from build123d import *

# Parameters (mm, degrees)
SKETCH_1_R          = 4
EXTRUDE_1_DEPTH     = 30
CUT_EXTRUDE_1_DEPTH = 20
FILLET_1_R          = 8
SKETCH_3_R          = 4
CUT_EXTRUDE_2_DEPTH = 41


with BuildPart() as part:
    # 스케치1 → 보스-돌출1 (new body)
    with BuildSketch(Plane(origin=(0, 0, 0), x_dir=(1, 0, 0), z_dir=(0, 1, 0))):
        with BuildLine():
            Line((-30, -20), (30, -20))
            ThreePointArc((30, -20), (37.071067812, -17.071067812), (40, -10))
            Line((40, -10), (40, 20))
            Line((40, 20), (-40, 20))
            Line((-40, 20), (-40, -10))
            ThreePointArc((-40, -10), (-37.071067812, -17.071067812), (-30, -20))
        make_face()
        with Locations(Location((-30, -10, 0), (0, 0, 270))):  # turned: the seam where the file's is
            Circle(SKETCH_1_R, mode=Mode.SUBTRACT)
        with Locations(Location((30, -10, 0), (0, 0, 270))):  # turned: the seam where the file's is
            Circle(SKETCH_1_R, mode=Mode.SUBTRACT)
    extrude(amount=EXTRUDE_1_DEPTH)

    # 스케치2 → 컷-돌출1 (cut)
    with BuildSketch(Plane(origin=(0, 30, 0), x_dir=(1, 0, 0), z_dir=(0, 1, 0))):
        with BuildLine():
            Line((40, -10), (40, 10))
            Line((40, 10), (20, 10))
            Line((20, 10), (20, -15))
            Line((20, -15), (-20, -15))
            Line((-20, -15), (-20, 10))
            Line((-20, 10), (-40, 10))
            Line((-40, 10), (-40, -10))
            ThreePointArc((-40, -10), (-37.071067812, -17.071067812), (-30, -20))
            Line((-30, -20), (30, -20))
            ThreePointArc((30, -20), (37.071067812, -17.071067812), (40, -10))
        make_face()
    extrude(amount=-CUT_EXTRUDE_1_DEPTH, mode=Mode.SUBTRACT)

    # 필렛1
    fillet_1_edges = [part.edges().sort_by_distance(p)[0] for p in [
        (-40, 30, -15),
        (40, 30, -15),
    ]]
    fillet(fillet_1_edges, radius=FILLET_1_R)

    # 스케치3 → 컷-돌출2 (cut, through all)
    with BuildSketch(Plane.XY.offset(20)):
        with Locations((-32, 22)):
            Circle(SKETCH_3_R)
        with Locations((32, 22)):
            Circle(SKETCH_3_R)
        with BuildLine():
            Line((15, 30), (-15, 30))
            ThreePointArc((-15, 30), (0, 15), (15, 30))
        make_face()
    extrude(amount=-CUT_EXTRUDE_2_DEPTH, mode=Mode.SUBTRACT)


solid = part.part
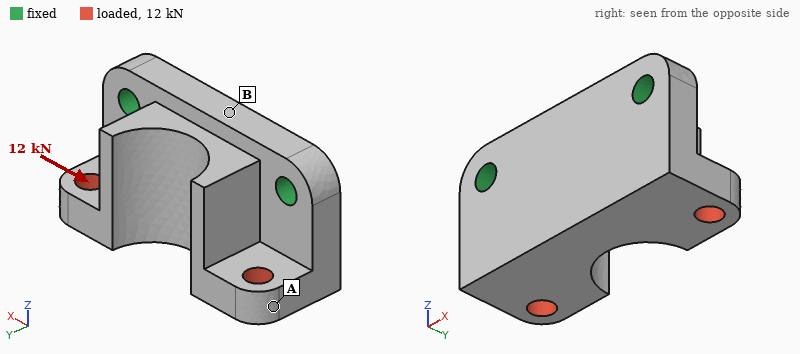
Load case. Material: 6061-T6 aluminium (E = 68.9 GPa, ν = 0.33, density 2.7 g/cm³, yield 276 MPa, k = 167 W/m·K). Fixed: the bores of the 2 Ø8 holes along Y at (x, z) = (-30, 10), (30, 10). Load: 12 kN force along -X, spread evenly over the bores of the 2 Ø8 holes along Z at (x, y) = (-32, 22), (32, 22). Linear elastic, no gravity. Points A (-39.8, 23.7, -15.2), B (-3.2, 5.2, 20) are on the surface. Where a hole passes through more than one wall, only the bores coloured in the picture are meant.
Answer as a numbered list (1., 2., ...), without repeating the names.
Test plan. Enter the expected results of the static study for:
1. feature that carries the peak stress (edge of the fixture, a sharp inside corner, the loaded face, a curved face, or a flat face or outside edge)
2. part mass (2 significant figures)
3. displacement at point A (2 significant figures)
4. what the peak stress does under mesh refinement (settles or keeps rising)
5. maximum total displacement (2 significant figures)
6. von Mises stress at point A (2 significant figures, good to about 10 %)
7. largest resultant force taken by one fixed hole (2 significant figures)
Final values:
1. edge of the fixture
2. 140 g
3. 70 µm
4. keeps rising
5. 71 µm
6. 43 MPa
7. 8.4 kN
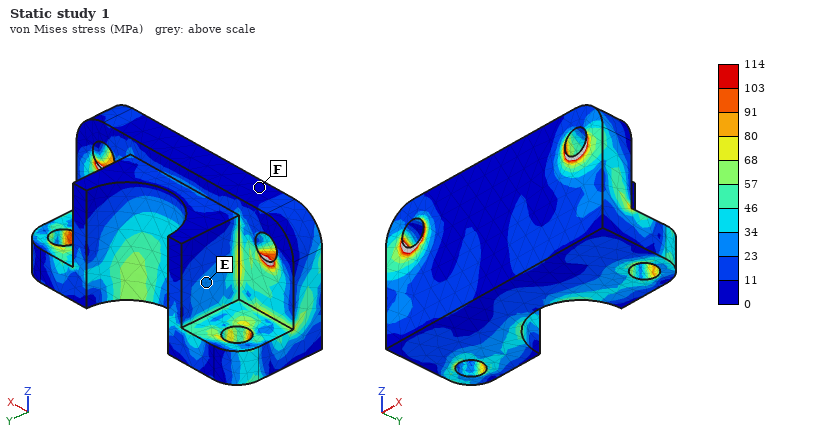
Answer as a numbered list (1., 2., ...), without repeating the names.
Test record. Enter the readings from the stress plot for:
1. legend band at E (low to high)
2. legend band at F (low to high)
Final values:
1. 23 to 34 MPa
2. 0 to 11 MPa
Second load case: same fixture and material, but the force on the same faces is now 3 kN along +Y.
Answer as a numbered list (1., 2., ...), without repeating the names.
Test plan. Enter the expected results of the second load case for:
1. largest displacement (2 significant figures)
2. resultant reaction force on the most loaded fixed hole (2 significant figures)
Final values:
1. 66 µm
2. 1.5 kN
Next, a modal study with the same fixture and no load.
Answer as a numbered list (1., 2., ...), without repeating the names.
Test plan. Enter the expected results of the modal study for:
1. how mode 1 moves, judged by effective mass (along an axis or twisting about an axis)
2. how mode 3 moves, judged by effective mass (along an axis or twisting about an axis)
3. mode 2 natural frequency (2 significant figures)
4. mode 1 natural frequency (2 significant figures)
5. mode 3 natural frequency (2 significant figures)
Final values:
1. along Y
2. along Y
3. 9000 Hz
4. 4500 Hz
5. 12 kHz
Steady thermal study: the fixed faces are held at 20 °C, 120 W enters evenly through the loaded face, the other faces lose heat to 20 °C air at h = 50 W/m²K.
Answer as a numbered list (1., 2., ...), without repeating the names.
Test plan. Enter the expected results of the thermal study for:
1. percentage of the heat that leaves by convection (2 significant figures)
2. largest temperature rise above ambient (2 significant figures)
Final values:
1. 8.9 %
2. 47 K
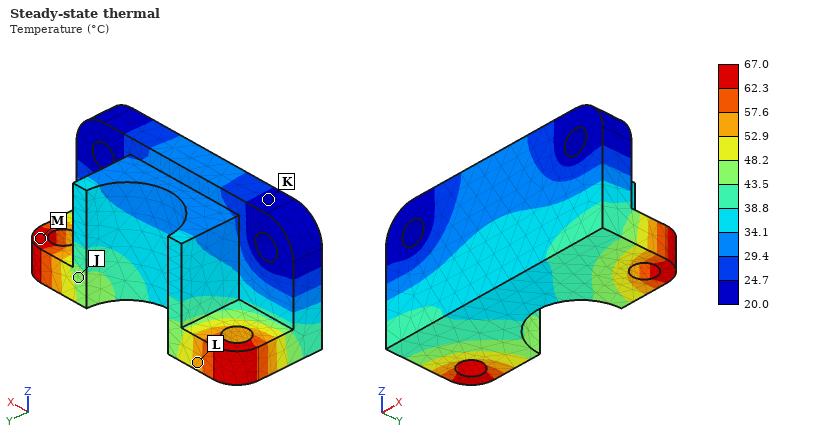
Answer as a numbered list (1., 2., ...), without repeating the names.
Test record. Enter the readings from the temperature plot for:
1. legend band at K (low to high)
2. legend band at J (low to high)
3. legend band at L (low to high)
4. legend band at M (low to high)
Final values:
1. 20.0 to 24.7 °C
2. 43.5 to 48.2 °C
3. 52.9 to 57.6 °C
4. 62.3 to 67.0 °C
